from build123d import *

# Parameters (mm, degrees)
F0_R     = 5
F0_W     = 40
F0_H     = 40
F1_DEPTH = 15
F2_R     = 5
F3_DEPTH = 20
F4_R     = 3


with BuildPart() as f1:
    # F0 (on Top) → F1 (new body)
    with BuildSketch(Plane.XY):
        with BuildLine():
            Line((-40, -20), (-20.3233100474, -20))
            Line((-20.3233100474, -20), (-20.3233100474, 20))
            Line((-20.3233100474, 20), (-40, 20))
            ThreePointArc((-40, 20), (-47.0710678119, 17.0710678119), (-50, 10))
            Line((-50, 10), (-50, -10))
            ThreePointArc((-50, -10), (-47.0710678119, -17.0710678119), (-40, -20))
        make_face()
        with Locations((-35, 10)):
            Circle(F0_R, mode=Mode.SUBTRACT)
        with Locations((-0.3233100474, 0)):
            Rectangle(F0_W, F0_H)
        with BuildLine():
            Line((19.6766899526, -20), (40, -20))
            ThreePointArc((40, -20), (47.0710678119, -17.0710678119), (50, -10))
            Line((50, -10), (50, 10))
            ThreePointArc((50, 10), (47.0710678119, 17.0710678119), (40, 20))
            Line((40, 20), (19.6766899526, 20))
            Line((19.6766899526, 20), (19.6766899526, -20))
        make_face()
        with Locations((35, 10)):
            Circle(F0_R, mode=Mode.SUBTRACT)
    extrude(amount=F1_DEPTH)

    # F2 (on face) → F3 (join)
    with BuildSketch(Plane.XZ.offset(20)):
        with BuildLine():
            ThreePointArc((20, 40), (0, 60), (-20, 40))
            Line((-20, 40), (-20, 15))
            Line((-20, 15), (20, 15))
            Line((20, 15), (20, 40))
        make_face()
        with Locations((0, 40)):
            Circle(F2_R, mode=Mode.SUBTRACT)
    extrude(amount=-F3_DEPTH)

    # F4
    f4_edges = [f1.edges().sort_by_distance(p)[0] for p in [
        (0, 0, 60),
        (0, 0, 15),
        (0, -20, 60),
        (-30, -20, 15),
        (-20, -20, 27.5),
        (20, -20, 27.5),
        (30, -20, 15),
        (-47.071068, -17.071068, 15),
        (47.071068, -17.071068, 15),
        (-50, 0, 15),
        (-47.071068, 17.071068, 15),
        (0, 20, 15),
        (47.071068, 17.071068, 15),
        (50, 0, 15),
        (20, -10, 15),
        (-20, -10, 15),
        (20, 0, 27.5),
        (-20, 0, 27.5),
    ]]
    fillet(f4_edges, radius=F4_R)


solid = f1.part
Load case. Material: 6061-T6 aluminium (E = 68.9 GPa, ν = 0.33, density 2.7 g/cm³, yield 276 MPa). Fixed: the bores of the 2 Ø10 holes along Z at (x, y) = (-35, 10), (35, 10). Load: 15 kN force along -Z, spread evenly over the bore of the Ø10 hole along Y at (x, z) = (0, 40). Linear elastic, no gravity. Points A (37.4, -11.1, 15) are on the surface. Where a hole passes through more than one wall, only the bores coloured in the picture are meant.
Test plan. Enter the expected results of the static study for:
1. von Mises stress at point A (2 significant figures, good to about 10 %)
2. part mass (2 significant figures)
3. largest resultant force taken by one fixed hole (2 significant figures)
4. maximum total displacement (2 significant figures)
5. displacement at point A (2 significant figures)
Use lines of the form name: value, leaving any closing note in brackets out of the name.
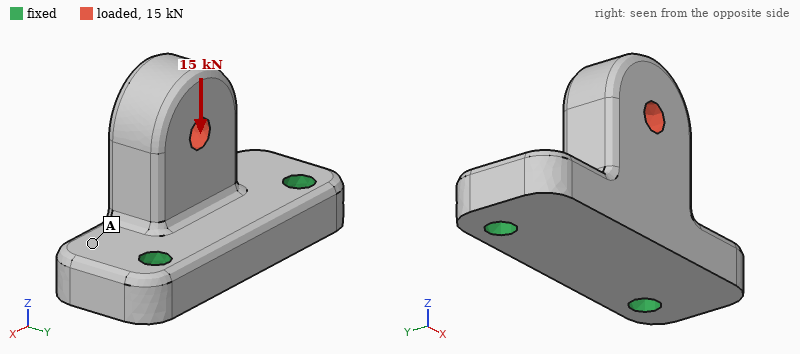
von Mises stress at point A: 30 MPa
part mass: 230 g
largest resultant force taken by one fixed hole: 7.6 kN
maximum total displacement: 0.19 mm
displacement at point A: 0.039 mm
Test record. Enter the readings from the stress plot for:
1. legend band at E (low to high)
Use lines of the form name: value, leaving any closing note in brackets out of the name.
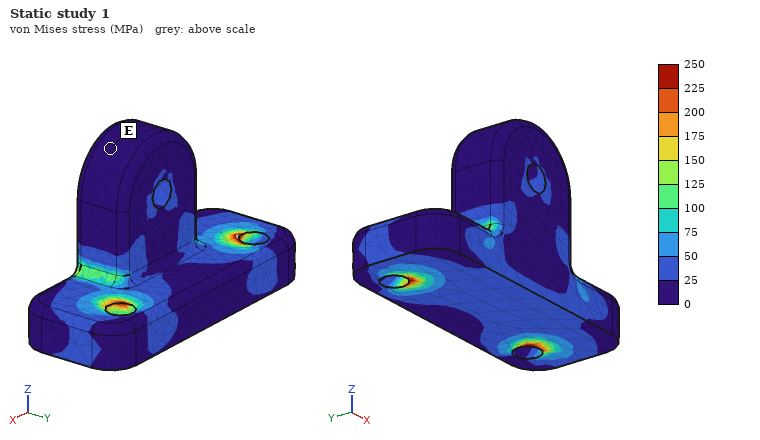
legend band at E: 0 to 25 MPa
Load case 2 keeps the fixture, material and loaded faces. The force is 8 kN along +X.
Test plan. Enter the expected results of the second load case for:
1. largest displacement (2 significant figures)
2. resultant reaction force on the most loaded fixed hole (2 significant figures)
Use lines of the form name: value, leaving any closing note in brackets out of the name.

largest displacement: 77 µm
resultant reaction force on the most loaded fixed hole: 6.2 kN
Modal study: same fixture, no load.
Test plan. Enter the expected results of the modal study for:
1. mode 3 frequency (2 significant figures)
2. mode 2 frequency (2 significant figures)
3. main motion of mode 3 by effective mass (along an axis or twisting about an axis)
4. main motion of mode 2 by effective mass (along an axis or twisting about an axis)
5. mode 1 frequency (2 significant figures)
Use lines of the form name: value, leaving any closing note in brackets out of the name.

mode 3 frequency: 8400 Hz
mode 2 frequency: 7000 Hz
main motion of mode 3 by effective mass: along Z
main motion of mode 2 by effective mass: along X
mode 1 frequency: 3500 Hz
